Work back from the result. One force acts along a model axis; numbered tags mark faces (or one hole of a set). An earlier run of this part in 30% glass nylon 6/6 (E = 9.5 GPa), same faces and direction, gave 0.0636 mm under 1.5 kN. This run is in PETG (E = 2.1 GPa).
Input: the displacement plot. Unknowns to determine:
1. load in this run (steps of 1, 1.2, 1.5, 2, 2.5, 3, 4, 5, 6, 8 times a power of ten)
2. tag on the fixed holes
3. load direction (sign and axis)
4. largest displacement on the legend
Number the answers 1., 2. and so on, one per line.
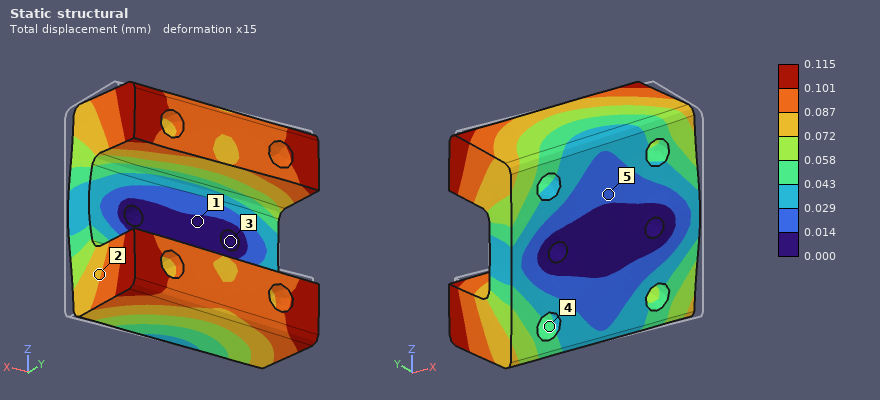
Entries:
1. 600 N
2. 3
3. -X
4. 0.115 mm
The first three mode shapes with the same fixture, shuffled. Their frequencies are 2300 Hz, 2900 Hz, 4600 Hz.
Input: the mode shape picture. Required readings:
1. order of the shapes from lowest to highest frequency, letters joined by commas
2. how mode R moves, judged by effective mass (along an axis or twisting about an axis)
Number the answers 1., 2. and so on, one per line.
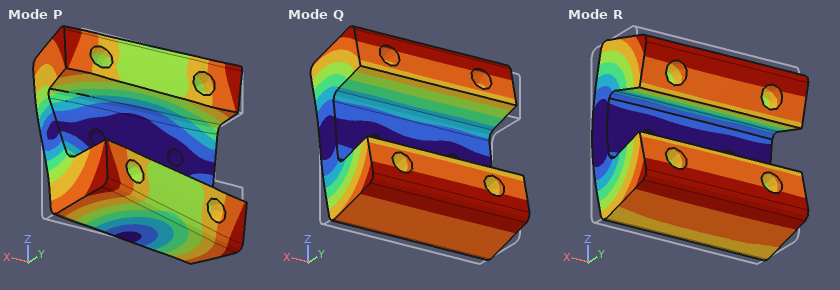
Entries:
1. Q, R, P
2. along Y
